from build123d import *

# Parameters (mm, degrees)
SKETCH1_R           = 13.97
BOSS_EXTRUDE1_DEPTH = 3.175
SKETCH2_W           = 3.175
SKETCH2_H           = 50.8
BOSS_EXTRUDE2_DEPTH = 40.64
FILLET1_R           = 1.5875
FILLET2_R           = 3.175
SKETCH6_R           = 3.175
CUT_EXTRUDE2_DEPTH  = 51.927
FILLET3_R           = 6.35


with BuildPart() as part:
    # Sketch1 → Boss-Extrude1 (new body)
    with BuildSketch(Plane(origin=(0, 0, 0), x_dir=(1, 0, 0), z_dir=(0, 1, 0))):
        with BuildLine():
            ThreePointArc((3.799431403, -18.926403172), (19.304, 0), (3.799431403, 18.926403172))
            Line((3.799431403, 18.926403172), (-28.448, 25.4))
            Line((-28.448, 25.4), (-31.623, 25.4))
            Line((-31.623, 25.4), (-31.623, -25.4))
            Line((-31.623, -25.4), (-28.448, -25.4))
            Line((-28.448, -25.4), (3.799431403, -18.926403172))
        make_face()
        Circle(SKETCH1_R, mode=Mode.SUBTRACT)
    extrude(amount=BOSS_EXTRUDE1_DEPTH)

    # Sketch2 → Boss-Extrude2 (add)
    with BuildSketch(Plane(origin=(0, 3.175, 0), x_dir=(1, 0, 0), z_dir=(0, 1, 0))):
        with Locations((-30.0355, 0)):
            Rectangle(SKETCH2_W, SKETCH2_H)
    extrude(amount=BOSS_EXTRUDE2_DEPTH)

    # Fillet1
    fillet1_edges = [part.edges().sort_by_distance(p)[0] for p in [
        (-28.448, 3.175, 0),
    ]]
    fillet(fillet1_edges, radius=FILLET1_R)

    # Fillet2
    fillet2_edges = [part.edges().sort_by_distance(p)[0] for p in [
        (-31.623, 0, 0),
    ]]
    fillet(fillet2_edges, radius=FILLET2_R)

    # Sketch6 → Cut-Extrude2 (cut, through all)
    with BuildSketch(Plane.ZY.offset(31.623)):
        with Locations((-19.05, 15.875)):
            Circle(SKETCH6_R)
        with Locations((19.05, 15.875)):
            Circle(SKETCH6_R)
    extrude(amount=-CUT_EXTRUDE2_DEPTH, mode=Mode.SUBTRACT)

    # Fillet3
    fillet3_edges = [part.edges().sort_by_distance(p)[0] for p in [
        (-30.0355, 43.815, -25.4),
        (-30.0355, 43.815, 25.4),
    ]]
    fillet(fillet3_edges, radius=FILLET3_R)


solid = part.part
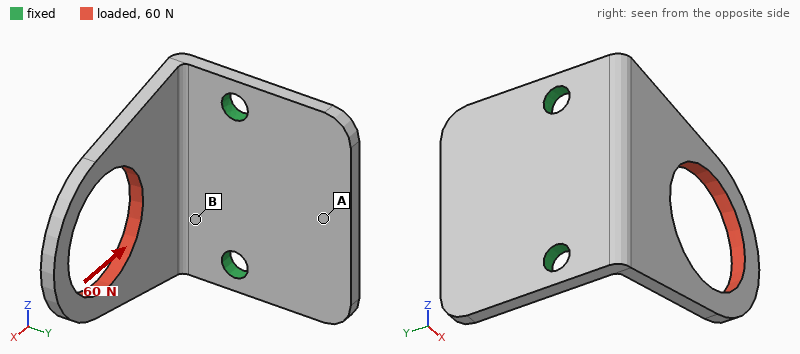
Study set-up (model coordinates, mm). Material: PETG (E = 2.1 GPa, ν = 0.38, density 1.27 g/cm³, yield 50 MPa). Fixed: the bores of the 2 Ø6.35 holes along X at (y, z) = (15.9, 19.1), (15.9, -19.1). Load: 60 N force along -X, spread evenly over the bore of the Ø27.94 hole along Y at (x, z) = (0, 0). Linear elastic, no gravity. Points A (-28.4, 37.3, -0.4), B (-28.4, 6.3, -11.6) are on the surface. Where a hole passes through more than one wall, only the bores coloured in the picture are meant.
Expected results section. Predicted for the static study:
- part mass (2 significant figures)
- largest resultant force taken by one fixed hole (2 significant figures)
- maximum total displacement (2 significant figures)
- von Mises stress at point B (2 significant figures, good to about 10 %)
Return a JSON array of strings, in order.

["14 g", "30 N", "0.87 mm", "3.1 MPa"]
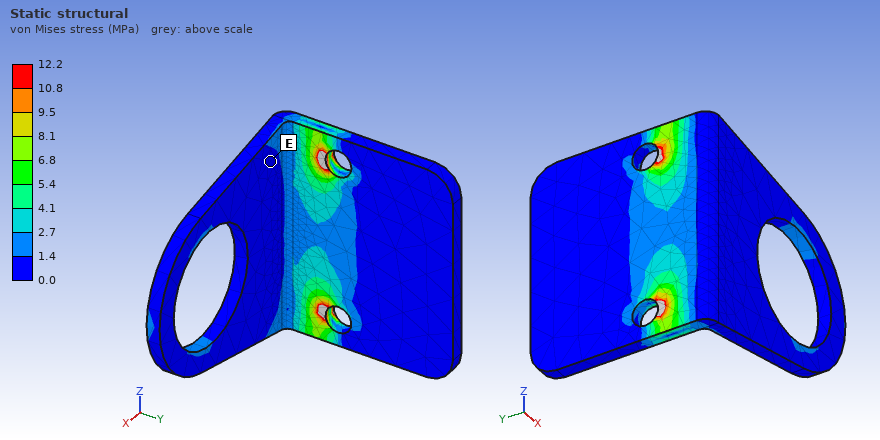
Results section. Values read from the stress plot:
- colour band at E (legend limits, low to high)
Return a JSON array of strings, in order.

["0.0 to 1.4 MPa"]
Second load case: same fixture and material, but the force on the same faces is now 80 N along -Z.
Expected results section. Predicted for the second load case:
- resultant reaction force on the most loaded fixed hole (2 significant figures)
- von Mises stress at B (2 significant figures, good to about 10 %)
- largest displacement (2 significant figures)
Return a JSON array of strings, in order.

["79 N", "6.7 MPa", "0.83 mm"]
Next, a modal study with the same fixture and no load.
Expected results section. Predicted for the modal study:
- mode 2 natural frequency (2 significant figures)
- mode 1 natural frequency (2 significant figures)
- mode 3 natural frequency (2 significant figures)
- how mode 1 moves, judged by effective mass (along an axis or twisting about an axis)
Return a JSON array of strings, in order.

["790 Hz", "320 Hz", "890 Hz", "along Y"]
